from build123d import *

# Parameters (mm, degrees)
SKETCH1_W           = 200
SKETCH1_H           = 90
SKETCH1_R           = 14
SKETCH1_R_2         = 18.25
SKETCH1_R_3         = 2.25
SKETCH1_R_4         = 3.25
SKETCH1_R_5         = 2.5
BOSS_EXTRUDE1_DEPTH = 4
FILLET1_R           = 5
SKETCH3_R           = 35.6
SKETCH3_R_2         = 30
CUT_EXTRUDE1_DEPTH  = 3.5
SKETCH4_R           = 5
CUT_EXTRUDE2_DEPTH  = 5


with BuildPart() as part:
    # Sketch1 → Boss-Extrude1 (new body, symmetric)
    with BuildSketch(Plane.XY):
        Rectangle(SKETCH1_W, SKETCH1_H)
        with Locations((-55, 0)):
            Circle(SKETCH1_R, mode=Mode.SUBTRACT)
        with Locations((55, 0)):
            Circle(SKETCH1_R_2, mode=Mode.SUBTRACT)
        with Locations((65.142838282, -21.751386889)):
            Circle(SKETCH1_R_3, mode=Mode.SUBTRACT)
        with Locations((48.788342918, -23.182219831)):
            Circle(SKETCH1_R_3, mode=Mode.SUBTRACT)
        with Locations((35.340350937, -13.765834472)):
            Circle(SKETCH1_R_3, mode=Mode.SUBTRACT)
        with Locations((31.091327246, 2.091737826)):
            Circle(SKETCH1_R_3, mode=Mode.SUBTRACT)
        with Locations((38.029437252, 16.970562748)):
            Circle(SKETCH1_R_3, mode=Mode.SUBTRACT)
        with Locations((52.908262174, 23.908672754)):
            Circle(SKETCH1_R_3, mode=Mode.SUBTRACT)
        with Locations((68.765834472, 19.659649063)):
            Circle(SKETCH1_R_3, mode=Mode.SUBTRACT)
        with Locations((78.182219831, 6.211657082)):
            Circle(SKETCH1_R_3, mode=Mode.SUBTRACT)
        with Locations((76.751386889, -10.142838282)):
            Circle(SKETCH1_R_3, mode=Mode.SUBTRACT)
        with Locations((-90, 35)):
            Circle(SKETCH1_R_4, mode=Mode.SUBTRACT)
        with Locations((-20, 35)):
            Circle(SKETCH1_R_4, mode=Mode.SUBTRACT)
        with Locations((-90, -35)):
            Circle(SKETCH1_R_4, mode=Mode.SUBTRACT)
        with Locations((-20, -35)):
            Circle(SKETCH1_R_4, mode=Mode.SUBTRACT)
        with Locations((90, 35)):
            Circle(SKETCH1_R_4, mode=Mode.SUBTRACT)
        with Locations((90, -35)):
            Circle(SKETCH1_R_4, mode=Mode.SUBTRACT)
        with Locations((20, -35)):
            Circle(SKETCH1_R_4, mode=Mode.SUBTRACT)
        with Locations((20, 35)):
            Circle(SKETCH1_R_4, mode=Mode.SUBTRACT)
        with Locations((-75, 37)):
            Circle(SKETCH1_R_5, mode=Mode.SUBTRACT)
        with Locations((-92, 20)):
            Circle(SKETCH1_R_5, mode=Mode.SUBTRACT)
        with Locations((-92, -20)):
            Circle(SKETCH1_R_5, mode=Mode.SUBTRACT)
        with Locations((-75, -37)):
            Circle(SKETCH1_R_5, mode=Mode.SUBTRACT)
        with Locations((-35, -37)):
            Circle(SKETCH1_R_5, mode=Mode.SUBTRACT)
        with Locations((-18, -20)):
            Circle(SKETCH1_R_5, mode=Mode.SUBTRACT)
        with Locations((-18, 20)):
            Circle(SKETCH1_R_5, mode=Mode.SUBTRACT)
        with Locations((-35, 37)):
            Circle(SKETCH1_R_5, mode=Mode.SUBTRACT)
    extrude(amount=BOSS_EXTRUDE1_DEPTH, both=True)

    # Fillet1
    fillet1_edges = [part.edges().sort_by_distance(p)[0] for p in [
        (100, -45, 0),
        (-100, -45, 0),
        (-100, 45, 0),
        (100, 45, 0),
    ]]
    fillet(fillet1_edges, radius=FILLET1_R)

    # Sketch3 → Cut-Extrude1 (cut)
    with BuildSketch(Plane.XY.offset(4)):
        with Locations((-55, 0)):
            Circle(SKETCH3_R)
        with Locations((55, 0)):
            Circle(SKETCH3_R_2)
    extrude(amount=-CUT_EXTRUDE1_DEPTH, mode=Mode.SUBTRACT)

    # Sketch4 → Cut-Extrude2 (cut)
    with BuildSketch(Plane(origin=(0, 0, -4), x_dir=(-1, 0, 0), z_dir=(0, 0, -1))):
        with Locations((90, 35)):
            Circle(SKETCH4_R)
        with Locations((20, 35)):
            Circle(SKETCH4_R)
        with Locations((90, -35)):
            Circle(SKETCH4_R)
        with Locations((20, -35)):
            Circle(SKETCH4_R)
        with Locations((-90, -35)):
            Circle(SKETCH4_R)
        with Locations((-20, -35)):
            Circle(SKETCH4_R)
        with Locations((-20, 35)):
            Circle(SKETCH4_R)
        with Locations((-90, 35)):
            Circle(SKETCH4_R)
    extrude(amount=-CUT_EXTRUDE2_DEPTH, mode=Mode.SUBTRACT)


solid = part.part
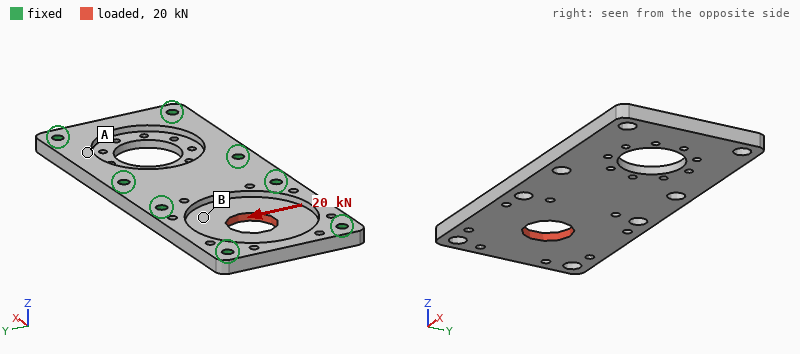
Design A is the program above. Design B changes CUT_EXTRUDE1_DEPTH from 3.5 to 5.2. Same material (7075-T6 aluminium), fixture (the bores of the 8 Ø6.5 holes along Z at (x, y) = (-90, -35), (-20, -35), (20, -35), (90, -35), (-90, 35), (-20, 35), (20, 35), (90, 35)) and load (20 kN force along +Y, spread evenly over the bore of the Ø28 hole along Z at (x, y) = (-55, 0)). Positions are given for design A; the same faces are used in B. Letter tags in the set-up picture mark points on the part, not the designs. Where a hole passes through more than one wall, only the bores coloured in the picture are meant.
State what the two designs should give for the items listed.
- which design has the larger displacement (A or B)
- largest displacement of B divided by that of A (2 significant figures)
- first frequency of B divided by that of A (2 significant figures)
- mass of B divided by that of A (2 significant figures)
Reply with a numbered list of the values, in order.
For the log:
1. B
2. 1.6
3. 0.97
4. 0.92
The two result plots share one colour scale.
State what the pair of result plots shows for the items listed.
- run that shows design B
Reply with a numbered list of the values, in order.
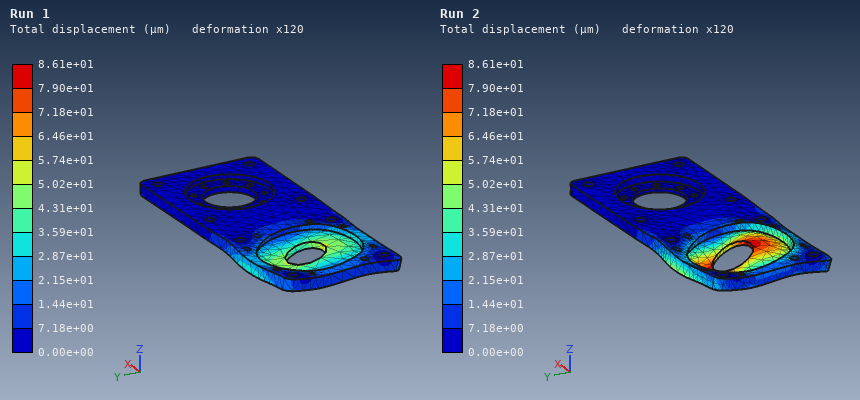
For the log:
1. Run 2
